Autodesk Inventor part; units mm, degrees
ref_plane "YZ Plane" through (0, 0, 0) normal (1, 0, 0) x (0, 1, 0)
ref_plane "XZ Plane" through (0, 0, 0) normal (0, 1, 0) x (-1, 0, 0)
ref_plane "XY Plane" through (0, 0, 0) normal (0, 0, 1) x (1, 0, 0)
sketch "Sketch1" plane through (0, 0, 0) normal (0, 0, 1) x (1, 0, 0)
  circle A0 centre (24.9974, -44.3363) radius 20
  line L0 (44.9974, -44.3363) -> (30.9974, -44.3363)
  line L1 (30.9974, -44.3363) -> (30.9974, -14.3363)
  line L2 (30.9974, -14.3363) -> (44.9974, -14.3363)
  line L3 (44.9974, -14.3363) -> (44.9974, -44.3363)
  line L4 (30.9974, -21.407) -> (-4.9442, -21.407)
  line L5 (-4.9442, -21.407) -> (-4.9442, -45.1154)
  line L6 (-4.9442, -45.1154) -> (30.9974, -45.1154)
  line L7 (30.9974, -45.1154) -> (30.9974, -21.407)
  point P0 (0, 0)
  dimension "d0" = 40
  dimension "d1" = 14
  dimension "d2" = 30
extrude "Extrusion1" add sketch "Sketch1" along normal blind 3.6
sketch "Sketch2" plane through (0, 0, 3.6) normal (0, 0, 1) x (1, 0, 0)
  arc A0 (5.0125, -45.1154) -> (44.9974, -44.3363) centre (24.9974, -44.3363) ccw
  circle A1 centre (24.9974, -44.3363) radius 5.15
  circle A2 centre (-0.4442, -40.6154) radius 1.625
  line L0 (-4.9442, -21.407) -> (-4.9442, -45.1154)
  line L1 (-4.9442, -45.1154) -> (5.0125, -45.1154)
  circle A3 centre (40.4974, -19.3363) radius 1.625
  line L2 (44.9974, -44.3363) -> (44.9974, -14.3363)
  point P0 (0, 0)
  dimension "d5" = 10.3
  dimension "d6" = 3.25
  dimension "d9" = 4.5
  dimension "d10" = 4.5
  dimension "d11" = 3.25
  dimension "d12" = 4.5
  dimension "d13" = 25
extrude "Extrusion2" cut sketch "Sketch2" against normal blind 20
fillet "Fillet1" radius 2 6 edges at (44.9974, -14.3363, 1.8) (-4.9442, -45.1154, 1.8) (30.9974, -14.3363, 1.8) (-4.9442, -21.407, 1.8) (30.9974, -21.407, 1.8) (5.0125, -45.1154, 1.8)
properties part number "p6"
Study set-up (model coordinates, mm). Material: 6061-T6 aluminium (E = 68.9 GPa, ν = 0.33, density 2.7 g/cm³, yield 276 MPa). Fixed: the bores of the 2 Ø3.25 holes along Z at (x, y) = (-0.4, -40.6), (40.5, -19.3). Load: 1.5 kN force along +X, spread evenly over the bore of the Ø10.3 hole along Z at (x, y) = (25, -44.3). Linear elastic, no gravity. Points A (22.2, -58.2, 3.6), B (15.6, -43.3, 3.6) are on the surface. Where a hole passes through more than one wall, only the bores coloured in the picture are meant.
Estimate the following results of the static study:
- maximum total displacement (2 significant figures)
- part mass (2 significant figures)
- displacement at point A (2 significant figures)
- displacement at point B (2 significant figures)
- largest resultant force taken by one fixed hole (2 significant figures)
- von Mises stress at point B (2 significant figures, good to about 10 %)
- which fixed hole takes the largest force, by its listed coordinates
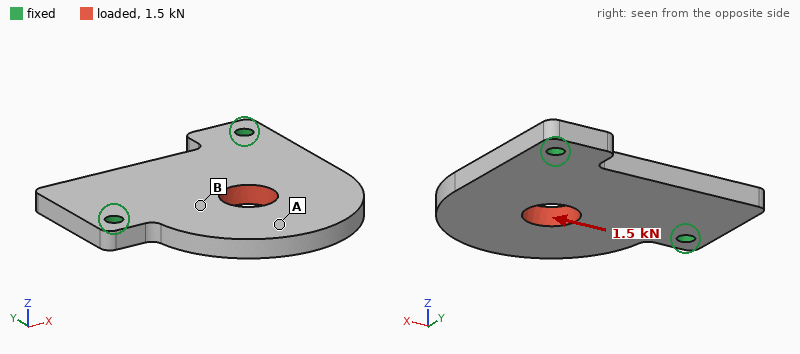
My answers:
13 µm
17 g
11 µm
6.2 µm
1.2 kN
21 MPa
(-0.4, -40.6)
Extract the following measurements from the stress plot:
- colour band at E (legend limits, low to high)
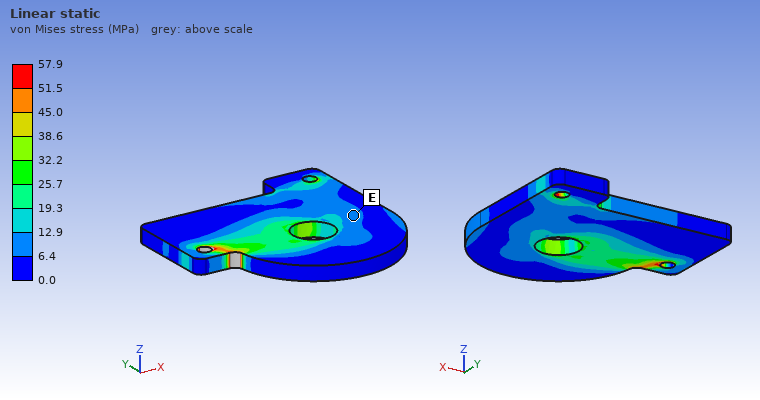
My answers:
6.4 to 12.9 MPa
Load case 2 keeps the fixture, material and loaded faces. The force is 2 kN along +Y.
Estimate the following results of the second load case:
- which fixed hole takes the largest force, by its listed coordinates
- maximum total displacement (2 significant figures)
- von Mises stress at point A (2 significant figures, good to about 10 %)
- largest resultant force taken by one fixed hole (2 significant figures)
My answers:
(40.5, -19.3)
13 µm
11 MPa
1.4 kN
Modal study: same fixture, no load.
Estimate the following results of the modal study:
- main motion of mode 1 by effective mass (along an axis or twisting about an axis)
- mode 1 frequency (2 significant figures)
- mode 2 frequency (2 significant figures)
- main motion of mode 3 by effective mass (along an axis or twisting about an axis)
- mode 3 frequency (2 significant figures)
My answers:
along Z
2200 Hz
6900 Hz
along Z
7500 Hz
